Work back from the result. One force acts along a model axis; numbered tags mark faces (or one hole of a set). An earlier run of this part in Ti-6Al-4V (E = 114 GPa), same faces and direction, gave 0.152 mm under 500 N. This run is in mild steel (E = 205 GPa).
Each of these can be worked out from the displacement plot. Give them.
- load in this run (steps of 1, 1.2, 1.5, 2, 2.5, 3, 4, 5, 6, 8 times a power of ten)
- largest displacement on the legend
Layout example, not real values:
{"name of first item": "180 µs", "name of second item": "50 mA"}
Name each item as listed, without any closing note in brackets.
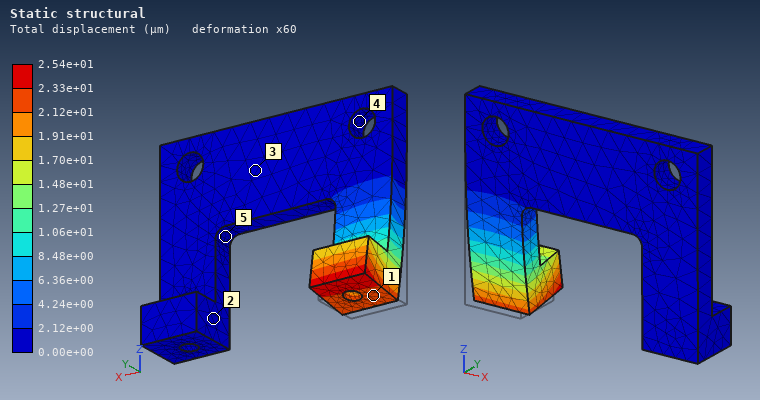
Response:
{"load in this run": "150 N", "largest displacement on the legend": "2.54e+01 µm"}
